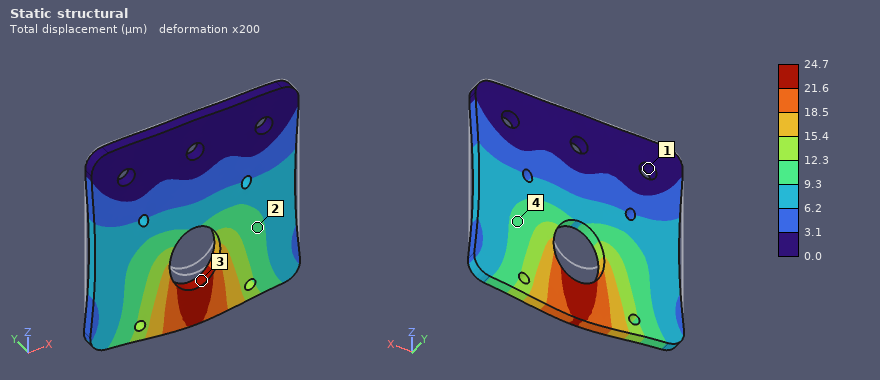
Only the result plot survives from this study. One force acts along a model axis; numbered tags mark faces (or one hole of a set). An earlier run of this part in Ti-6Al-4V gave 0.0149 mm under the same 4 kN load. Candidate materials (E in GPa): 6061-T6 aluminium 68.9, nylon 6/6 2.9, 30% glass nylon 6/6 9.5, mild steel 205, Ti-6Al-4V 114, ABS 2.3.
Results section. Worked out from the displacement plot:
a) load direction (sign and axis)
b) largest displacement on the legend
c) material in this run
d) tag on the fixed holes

-Z
24.7 µm
6061-T6 aluminium
1
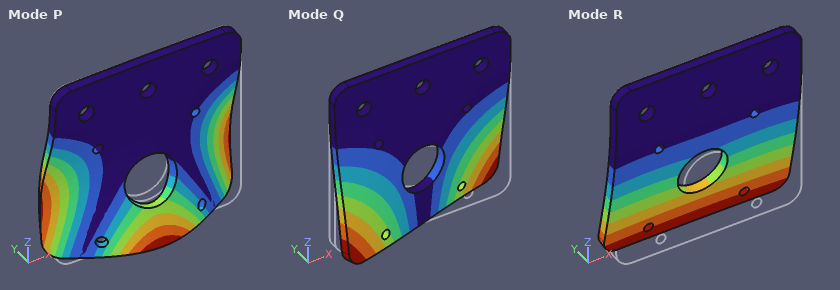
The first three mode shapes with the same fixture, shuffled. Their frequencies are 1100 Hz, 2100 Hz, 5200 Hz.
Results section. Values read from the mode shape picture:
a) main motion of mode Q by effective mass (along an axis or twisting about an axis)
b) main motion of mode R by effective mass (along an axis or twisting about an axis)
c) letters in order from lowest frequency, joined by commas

twisting about Z
along Y
R, Q, P
